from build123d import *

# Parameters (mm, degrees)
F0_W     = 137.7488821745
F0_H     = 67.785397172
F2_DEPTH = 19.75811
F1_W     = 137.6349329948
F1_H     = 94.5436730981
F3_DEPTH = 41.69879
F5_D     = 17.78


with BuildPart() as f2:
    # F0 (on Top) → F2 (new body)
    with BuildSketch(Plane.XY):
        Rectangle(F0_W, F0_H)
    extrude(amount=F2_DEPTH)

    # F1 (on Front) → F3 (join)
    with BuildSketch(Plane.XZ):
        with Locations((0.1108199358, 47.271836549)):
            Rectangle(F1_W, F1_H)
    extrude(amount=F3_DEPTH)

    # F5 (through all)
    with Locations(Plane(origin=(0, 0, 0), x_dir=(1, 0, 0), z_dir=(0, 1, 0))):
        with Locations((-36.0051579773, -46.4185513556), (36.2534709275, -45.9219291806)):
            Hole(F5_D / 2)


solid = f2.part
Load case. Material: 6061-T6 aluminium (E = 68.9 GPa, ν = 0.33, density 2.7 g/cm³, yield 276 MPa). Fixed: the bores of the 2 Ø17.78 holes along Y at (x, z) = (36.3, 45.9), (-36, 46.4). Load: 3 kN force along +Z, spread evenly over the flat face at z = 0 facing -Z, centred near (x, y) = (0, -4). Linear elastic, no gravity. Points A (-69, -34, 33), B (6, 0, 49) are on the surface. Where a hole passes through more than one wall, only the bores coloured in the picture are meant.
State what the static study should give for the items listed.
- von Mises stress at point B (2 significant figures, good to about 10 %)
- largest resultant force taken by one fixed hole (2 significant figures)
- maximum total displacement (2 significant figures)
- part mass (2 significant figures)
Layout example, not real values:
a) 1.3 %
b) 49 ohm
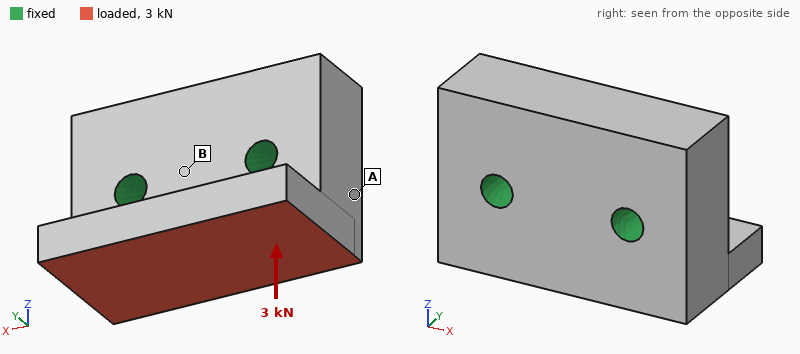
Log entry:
a) 0.66 MPa
b) 1.5 kN
c) 5.1 µm
d) 1.7 kg
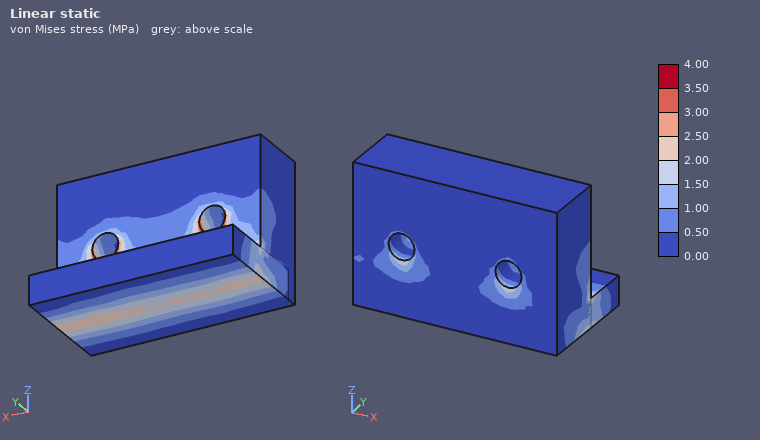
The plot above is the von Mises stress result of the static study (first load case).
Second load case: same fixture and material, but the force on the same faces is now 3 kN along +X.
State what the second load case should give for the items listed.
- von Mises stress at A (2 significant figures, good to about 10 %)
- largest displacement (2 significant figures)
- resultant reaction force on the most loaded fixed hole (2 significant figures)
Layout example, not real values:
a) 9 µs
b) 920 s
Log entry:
a) 0.82 MPa
b) 3.1 µm
c) 2.2 kN
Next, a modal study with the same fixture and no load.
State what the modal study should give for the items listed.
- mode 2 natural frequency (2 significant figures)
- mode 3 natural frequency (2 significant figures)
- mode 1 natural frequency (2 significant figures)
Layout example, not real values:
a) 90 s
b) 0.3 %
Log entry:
a) 7100 Hz
b) 8500 Hz
c) 5700 Hz
